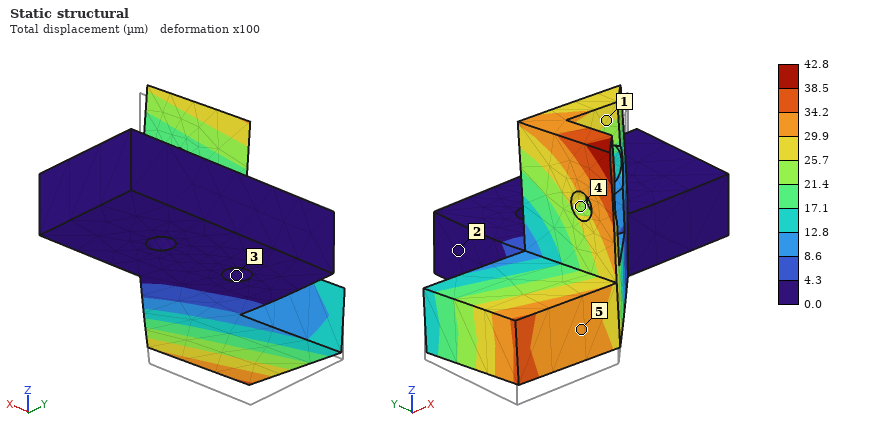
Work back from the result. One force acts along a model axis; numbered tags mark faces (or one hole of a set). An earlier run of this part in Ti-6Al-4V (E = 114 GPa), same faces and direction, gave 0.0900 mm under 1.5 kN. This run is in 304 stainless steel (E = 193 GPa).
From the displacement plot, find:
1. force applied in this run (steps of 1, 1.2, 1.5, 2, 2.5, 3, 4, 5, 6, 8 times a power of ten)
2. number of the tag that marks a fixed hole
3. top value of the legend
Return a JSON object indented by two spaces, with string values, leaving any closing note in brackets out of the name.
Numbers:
{
  "force applied in this run": "1.2 kN",
  "number of the tag that marks a fixed hole": "3",
  "top value of the legend": "42.8 µm"
}
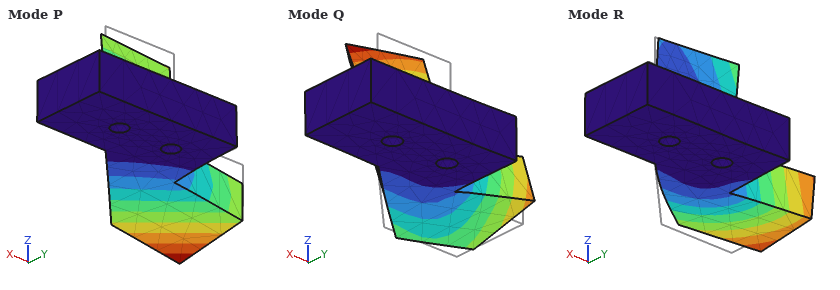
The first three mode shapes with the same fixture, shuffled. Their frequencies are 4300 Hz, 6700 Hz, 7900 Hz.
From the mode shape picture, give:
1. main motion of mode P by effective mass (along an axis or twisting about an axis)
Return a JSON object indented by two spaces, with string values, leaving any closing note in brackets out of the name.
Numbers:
{
  "main motion of mode P by effective mass": "along Z"
}
